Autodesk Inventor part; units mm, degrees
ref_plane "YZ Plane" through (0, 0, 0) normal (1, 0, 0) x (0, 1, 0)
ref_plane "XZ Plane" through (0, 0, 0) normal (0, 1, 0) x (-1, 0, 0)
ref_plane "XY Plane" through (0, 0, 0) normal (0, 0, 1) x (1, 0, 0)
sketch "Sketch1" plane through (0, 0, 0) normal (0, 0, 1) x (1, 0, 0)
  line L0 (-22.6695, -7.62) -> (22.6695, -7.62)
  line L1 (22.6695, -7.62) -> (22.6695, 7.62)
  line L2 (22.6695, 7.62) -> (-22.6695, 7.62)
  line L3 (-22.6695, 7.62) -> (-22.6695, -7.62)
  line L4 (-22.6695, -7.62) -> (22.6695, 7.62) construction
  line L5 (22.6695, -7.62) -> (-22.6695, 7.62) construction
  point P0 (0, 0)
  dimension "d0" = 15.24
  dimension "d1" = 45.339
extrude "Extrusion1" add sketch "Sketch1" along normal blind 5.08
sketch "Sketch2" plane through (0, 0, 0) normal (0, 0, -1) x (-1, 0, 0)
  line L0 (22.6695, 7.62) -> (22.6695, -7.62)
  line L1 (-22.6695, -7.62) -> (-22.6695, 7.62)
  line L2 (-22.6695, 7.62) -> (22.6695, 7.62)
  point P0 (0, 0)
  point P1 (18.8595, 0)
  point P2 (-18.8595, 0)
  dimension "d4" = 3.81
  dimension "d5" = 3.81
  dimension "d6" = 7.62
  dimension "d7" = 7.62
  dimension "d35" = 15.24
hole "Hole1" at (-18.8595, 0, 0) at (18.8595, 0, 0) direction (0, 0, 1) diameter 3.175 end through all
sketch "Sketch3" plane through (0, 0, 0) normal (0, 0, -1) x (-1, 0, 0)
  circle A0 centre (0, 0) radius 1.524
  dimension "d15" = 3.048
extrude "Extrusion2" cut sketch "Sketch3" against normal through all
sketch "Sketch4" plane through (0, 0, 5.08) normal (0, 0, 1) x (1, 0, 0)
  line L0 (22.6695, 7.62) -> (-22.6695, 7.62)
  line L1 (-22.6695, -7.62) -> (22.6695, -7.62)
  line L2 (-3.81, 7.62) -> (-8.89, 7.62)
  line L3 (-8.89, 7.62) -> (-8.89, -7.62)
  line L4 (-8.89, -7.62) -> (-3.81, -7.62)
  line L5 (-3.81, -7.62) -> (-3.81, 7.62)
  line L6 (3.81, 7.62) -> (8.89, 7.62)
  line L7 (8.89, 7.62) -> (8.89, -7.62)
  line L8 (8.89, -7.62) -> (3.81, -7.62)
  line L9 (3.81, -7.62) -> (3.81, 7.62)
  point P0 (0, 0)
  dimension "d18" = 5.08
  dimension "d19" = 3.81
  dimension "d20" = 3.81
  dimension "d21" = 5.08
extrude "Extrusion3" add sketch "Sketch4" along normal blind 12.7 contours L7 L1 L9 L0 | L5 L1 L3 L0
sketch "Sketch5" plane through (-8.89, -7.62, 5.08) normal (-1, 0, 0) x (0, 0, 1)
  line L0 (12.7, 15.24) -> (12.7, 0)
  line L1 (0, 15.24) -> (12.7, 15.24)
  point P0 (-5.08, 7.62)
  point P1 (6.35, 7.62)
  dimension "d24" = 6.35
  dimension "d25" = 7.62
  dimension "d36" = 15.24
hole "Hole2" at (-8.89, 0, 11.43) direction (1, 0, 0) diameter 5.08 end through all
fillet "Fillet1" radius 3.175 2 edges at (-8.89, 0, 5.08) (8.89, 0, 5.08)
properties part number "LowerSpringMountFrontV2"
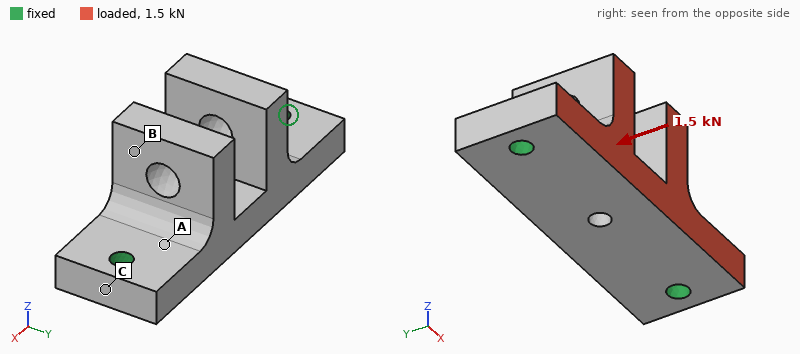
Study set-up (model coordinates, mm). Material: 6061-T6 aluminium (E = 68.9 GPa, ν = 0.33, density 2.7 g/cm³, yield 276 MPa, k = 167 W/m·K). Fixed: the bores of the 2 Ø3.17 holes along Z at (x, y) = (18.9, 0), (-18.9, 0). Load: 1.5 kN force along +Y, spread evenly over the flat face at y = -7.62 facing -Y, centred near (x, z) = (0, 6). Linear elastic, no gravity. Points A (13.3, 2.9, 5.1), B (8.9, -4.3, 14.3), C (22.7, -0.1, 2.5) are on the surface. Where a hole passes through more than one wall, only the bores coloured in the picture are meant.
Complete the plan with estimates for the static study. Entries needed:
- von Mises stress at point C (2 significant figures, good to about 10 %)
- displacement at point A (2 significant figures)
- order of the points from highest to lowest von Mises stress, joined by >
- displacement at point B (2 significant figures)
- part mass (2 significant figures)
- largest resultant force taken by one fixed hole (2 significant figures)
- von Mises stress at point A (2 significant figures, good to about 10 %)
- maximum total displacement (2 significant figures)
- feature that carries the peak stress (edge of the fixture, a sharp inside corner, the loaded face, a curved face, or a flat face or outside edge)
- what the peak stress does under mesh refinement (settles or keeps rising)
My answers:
17 MPa
7.5 µm
A > C > B
30 µm
14 g
750 N
43 MPa
39 µm
edge of the fixture
keeps rising
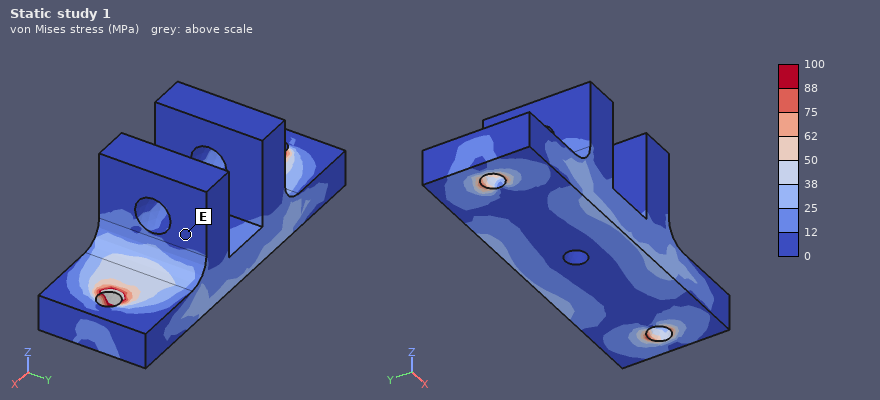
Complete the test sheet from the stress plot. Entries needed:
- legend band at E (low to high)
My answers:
0 to 12 MPa
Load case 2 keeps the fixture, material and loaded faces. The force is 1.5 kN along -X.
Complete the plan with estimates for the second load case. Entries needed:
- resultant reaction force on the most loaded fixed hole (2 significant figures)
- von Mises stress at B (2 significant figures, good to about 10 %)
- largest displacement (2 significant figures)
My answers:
820 N
10.0 MPa
22 µm
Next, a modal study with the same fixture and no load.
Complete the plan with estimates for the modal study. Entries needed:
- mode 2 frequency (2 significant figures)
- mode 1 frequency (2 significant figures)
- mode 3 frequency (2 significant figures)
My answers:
10000 Hz
9700 Hz
18 kHz
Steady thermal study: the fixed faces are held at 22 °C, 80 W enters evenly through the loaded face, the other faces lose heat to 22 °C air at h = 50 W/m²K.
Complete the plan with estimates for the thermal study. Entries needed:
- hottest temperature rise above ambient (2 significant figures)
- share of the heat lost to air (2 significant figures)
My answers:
43 K
4.0 %
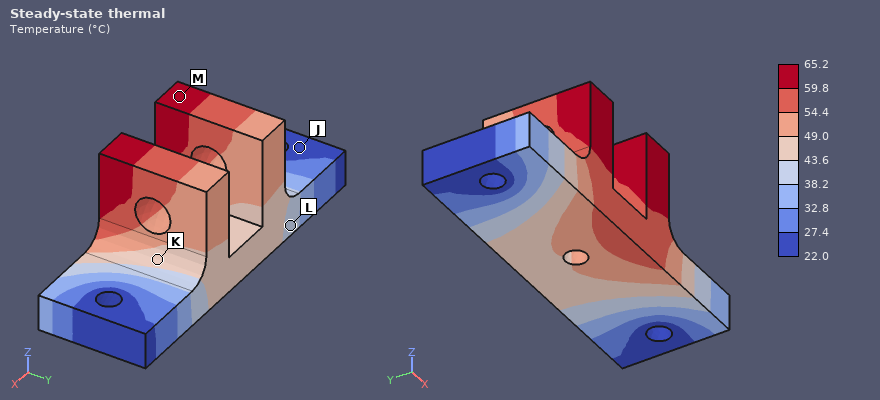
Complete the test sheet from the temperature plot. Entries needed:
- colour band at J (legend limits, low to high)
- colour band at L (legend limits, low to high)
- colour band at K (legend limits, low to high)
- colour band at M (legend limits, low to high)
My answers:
22.0 to 27.4 °C
38.2 to 43.6 °C
43.6 to 49.0 °C
59.8 to 65.2 °C
